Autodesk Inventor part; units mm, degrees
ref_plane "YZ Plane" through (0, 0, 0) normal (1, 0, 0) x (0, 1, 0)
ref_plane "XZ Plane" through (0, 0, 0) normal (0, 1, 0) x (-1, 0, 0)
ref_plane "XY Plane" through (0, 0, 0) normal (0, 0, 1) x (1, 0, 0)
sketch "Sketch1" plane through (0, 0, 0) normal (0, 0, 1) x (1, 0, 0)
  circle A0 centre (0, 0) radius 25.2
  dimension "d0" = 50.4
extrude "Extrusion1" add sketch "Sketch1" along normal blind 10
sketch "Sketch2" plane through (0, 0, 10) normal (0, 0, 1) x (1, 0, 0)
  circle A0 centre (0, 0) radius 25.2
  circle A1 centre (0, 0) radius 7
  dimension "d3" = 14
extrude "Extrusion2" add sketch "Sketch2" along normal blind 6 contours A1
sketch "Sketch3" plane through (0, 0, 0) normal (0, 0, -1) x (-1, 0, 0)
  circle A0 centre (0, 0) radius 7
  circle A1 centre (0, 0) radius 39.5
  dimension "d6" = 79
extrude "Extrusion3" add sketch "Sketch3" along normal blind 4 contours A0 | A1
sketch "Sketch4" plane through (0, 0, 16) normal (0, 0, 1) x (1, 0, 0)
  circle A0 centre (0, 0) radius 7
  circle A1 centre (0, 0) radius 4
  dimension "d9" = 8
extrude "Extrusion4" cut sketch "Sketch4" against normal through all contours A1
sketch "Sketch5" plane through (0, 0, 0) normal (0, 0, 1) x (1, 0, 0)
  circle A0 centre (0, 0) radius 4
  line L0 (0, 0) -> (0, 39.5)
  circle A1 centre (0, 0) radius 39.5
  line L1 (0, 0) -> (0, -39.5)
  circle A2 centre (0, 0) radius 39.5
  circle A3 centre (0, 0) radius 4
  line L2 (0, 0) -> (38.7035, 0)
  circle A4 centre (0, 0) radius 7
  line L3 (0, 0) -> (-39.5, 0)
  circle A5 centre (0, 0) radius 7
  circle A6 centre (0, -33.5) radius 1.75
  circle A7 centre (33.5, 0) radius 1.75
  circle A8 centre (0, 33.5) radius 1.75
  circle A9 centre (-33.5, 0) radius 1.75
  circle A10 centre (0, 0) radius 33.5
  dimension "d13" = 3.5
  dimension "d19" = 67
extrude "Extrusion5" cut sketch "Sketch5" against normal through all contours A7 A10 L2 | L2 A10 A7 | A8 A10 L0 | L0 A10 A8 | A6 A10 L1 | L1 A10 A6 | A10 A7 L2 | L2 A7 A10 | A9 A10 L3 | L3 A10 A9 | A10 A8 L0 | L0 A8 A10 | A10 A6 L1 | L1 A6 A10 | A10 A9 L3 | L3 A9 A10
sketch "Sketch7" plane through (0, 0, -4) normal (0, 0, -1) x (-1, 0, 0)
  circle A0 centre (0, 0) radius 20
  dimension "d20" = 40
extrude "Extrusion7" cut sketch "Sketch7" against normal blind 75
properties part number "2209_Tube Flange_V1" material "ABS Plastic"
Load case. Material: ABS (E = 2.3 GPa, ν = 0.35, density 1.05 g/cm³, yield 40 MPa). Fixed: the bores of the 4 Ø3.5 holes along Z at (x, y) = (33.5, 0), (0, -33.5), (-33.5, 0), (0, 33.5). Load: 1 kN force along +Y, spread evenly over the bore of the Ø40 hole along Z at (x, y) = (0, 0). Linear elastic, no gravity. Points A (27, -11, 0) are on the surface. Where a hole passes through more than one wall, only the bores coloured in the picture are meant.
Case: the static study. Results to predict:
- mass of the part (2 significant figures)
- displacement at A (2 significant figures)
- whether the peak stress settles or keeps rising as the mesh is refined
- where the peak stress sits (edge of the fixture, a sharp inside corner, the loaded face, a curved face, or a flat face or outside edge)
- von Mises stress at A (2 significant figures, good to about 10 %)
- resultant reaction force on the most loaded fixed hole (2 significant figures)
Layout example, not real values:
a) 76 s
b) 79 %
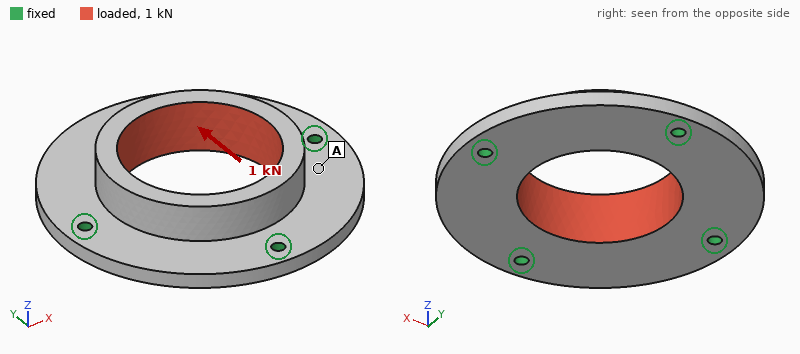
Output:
a) 23 g
b) 37 µm
c) keeps rising
d) edge of the fixture
e) 2.0 MPa
f) 260 N
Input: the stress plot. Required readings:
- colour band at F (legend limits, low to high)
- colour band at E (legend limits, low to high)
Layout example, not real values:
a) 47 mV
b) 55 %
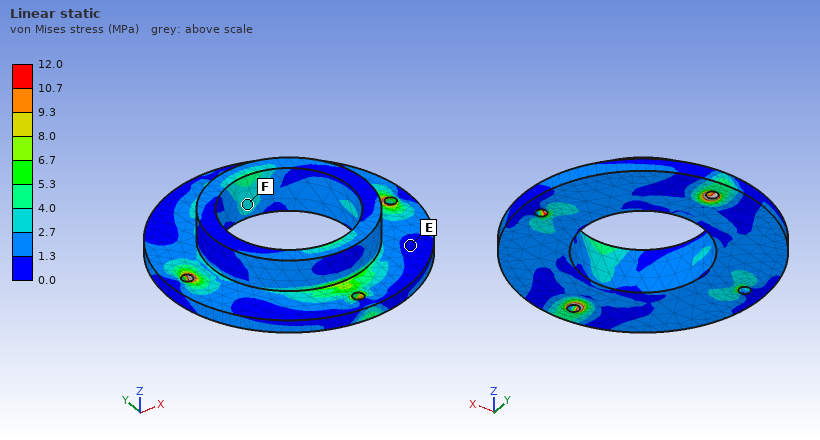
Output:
a) 2.7 to 4.0 MPa
b) 0.0 to 1.3 MPa
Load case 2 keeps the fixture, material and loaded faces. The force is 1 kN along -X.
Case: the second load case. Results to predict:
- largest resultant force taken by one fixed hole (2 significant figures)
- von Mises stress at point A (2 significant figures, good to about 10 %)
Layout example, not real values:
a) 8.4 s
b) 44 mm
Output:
a) 260 N
b) 3.7 MPa
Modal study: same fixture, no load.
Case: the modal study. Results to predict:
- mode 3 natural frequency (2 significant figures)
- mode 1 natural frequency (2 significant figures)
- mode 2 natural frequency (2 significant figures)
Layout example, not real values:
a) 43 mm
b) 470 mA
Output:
a) 2500 Hz
b) 2300 Hz
c) 2500 Hz
